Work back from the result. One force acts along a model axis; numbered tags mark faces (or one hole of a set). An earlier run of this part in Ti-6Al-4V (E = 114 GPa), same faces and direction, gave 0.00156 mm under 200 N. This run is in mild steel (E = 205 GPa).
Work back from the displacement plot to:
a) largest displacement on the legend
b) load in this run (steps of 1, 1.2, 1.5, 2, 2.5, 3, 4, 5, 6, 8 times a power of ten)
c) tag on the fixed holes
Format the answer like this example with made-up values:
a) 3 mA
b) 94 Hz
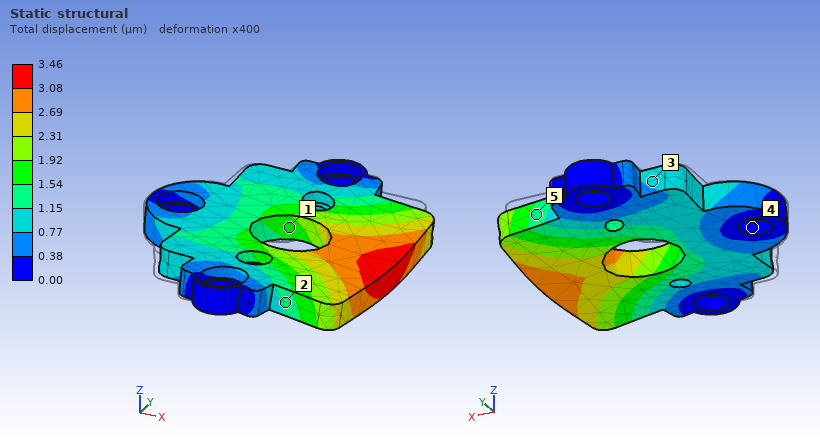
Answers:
a) 3.46 µm
b) 800 N
c) 4
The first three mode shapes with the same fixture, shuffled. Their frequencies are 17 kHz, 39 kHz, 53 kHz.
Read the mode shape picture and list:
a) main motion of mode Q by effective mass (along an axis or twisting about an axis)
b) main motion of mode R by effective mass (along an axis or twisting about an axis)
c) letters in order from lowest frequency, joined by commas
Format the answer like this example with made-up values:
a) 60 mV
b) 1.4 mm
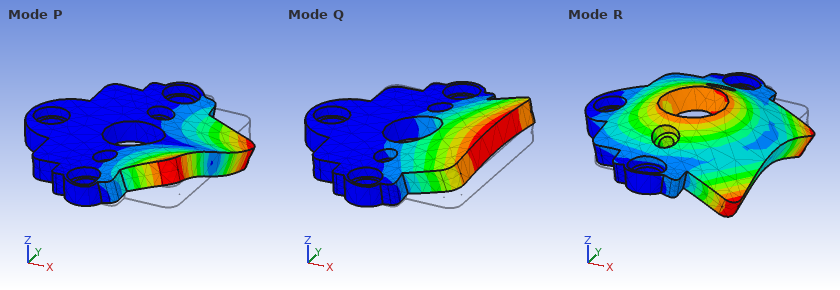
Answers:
a) along Z
b) along Z
c) Q, P, R
